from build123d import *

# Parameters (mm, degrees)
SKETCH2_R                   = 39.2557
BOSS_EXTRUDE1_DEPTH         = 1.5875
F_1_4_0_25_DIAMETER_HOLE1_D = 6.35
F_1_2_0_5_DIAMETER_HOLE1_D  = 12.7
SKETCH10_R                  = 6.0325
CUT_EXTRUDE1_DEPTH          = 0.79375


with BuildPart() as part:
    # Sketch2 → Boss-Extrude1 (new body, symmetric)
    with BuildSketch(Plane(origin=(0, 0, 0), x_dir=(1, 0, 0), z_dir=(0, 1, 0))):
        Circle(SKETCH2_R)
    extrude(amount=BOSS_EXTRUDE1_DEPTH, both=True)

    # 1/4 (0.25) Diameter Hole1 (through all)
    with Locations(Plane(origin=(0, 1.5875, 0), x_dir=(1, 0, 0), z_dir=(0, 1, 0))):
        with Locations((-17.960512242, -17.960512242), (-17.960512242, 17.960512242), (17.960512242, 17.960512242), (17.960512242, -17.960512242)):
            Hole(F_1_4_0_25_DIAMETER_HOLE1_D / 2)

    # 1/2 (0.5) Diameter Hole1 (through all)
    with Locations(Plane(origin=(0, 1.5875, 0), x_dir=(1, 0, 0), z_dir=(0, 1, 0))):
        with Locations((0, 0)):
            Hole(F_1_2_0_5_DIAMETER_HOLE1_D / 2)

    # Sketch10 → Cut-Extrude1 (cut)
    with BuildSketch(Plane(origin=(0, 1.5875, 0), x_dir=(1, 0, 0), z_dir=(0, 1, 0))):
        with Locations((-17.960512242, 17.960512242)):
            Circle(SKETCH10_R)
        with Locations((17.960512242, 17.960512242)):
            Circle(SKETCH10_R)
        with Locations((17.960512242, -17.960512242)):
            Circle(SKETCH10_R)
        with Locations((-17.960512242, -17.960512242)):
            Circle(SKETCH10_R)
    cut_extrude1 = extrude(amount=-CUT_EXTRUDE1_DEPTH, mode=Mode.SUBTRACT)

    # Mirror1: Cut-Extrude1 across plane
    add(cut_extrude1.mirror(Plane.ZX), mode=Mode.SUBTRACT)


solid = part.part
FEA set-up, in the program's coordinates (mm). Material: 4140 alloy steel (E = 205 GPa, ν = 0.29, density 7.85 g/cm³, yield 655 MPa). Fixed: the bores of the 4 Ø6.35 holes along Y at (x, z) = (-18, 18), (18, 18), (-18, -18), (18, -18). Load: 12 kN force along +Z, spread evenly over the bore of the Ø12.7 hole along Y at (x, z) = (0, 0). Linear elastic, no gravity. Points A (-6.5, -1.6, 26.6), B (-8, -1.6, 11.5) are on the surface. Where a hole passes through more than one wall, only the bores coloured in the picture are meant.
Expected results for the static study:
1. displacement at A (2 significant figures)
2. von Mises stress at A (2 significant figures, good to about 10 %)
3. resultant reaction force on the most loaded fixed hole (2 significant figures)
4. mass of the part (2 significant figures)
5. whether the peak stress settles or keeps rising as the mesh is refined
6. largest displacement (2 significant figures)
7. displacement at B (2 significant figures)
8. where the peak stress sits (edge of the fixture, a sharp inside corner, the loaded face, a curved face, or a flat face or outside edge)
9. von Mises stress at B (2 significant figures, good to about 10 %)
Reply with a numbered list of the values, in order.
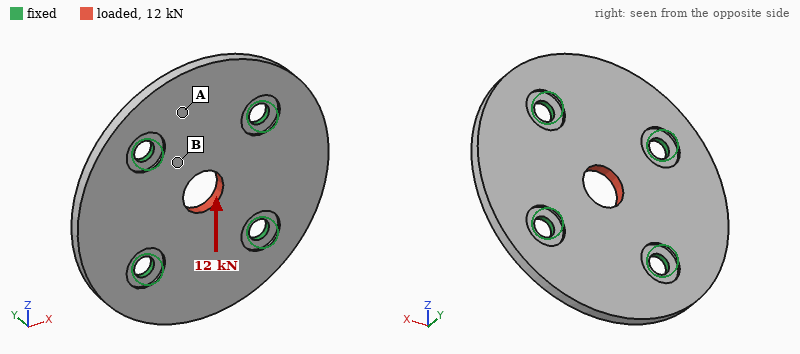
1. 4.1 µm
2. 26 MPa
3. 3.1 kN
4. 110 g
5. keeps rising
6. 9.4 µm
7. 5.4 µm
8. edge of the fixture
9. 66 MPa
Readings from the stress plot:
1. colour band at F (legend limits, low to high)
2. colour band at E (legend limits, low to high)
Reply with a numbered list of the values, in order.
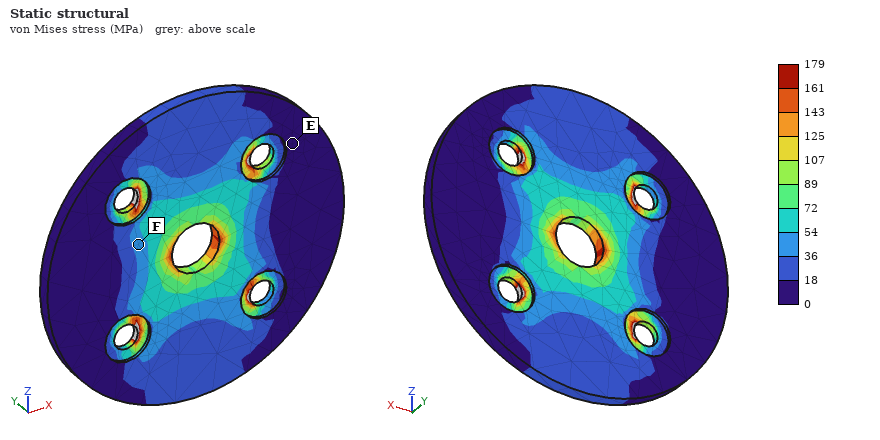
1. 36 to 54 MPa
2. 0 to 18 MPa
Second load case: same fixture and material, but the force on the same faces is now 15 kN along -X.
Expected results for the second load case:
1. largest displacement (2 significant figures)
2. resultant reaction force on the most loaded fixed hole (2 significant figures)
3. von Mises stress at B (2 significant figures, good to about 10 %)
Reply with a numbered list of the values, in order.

1. 12 µm
2. 3.9 kN
3. 78 MPa
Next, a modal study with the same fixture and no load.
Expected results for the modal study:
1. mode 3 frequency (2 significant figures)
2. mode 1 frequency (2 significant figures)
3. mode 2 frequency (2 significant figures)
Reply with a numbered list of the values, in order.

1. 5000 Hz
2. 4500 Hz
3. 5000 Hz
